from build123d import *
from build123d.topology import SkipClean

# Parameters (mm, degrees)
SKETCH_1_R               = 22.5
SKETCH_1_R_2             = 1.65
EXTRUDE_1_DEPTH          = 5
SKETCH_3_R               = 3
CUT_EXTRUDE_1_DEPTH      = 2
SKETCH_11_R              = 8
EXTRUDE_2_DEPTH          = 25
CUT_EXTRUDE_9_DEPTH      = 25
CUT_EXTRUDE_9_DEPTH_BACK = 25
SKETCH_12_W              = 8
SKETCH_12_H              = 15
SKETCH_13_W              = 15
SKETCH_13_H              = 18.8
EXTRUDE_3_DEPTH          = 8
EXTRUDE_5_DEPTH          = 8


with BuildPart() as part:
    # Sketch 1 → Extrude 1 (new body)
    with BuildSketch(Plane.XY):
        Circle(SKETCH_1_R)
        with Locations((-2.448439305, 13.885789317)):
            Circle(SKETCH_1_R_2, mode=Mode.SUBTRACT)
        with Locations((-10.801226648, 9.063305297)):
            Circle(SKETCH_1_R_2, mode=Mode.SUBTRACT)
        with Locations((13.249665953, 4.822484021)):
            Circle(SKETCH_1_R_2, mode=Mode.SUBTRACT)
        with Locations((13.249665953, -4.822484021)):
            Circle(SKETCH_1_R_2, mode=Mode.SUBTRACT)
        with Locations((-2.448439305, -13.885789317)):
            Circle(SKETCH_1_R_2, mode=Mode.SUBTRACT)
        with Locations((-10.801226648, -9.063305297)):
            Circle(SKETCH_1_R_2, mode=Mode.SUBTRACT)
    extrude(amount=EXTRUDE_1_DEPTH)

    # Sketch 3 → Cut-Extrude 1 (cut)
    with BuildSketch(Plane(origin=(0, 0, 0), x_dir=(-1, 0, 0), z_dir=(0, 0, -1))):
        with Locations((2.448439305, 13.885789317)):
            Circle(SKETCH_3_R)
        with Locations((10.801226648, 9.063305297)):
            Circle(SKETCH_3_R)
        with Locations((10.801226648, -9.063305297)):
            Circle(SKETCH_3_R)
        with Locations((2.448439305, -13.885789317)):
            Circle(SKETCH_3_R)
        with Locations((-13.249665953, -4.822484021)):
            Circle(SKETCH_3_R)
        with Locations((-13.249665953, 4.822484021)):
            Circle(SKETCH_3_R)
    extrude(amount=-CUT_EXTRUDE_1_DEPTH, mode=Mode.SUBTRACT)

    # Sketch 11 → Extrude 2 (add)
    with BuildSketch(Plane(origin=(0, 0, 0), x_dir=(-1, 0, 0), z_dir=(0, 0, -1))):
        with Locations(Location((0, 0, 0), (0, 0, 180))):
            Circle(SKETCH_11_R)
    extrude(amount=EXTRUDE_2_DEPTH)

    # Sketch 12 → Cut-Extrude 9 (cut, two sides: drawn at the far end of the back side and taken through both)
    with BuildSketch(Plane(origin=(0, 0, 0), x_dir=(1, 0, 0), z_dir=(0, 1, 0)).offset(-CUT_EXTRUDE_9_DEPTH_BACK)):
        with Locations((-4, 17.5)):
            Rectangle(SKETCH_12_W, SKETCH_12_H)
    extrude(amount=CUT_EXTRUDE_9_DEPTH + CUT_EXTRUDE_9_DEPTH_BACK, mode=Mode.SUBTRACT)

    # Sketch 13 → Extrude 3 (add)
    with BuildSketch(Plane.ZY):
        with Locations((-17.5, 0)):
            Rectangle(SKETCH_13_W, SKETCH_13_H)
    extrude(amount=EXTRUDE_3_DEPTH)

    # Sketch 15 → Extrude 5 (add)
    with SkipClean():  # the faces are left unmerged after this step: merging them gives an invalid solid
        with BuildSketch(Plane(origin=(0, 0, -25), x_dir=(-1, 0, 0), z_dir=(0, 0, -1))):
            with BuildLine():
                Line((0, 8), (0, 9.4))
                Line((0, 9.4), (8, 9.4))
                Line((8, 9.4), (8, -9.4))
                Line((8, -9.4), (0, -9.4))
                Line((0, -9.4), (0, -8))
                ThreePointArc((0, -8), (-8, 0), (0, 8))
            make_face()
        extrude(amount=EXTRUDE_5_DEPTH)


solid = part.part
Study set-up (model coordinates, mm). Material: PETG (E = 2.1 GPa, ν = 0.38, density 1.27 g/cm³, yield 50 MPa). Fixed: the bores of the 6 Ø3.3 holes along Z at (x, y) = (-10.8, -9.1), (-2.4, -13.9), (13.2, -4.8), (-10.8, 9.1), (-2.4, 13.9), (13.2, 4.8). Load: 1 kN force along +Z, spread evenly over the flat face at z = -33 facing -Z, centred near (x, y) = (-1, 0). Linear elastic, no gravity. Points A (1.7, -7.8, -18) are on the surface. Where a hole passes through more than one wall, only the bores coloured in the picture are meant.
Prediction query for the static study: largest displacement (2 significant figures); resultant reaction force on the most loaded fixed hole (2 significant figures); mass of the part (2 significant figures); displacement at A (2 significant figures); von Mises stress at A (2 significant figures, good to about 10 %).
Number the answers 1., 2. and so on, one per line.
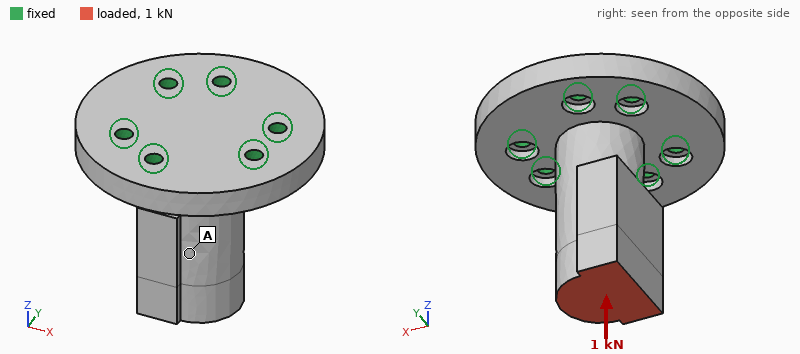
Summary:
1. 0.20 mm
2. 230 N
3. 19 g
4. 0.12 mm
5. 4.1 MPa
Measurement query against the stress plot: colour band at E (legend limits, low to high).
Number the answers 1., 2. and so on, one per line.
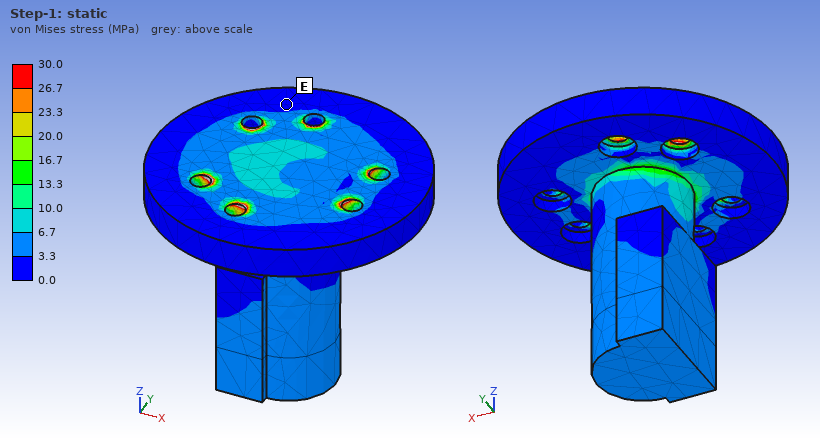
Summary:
1. 0.0 to 3.3 MPa
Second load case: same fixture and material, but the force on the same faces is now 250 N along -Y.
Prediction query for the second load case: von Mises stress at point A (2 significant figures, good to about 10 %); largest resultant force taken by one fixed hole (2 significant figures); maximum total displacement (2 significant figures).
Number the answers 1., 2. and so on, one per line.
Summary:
1. 6.3 MPa
2. 260 N
3. 0.86 mm
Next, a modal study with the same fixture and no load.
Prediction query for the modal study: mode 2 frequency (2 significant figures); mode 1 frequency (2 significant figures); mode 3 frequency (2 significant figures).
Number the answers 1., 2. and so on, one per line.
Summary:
1. 1500 Hz
2. 1500 Hz
3. 4500 Hz
